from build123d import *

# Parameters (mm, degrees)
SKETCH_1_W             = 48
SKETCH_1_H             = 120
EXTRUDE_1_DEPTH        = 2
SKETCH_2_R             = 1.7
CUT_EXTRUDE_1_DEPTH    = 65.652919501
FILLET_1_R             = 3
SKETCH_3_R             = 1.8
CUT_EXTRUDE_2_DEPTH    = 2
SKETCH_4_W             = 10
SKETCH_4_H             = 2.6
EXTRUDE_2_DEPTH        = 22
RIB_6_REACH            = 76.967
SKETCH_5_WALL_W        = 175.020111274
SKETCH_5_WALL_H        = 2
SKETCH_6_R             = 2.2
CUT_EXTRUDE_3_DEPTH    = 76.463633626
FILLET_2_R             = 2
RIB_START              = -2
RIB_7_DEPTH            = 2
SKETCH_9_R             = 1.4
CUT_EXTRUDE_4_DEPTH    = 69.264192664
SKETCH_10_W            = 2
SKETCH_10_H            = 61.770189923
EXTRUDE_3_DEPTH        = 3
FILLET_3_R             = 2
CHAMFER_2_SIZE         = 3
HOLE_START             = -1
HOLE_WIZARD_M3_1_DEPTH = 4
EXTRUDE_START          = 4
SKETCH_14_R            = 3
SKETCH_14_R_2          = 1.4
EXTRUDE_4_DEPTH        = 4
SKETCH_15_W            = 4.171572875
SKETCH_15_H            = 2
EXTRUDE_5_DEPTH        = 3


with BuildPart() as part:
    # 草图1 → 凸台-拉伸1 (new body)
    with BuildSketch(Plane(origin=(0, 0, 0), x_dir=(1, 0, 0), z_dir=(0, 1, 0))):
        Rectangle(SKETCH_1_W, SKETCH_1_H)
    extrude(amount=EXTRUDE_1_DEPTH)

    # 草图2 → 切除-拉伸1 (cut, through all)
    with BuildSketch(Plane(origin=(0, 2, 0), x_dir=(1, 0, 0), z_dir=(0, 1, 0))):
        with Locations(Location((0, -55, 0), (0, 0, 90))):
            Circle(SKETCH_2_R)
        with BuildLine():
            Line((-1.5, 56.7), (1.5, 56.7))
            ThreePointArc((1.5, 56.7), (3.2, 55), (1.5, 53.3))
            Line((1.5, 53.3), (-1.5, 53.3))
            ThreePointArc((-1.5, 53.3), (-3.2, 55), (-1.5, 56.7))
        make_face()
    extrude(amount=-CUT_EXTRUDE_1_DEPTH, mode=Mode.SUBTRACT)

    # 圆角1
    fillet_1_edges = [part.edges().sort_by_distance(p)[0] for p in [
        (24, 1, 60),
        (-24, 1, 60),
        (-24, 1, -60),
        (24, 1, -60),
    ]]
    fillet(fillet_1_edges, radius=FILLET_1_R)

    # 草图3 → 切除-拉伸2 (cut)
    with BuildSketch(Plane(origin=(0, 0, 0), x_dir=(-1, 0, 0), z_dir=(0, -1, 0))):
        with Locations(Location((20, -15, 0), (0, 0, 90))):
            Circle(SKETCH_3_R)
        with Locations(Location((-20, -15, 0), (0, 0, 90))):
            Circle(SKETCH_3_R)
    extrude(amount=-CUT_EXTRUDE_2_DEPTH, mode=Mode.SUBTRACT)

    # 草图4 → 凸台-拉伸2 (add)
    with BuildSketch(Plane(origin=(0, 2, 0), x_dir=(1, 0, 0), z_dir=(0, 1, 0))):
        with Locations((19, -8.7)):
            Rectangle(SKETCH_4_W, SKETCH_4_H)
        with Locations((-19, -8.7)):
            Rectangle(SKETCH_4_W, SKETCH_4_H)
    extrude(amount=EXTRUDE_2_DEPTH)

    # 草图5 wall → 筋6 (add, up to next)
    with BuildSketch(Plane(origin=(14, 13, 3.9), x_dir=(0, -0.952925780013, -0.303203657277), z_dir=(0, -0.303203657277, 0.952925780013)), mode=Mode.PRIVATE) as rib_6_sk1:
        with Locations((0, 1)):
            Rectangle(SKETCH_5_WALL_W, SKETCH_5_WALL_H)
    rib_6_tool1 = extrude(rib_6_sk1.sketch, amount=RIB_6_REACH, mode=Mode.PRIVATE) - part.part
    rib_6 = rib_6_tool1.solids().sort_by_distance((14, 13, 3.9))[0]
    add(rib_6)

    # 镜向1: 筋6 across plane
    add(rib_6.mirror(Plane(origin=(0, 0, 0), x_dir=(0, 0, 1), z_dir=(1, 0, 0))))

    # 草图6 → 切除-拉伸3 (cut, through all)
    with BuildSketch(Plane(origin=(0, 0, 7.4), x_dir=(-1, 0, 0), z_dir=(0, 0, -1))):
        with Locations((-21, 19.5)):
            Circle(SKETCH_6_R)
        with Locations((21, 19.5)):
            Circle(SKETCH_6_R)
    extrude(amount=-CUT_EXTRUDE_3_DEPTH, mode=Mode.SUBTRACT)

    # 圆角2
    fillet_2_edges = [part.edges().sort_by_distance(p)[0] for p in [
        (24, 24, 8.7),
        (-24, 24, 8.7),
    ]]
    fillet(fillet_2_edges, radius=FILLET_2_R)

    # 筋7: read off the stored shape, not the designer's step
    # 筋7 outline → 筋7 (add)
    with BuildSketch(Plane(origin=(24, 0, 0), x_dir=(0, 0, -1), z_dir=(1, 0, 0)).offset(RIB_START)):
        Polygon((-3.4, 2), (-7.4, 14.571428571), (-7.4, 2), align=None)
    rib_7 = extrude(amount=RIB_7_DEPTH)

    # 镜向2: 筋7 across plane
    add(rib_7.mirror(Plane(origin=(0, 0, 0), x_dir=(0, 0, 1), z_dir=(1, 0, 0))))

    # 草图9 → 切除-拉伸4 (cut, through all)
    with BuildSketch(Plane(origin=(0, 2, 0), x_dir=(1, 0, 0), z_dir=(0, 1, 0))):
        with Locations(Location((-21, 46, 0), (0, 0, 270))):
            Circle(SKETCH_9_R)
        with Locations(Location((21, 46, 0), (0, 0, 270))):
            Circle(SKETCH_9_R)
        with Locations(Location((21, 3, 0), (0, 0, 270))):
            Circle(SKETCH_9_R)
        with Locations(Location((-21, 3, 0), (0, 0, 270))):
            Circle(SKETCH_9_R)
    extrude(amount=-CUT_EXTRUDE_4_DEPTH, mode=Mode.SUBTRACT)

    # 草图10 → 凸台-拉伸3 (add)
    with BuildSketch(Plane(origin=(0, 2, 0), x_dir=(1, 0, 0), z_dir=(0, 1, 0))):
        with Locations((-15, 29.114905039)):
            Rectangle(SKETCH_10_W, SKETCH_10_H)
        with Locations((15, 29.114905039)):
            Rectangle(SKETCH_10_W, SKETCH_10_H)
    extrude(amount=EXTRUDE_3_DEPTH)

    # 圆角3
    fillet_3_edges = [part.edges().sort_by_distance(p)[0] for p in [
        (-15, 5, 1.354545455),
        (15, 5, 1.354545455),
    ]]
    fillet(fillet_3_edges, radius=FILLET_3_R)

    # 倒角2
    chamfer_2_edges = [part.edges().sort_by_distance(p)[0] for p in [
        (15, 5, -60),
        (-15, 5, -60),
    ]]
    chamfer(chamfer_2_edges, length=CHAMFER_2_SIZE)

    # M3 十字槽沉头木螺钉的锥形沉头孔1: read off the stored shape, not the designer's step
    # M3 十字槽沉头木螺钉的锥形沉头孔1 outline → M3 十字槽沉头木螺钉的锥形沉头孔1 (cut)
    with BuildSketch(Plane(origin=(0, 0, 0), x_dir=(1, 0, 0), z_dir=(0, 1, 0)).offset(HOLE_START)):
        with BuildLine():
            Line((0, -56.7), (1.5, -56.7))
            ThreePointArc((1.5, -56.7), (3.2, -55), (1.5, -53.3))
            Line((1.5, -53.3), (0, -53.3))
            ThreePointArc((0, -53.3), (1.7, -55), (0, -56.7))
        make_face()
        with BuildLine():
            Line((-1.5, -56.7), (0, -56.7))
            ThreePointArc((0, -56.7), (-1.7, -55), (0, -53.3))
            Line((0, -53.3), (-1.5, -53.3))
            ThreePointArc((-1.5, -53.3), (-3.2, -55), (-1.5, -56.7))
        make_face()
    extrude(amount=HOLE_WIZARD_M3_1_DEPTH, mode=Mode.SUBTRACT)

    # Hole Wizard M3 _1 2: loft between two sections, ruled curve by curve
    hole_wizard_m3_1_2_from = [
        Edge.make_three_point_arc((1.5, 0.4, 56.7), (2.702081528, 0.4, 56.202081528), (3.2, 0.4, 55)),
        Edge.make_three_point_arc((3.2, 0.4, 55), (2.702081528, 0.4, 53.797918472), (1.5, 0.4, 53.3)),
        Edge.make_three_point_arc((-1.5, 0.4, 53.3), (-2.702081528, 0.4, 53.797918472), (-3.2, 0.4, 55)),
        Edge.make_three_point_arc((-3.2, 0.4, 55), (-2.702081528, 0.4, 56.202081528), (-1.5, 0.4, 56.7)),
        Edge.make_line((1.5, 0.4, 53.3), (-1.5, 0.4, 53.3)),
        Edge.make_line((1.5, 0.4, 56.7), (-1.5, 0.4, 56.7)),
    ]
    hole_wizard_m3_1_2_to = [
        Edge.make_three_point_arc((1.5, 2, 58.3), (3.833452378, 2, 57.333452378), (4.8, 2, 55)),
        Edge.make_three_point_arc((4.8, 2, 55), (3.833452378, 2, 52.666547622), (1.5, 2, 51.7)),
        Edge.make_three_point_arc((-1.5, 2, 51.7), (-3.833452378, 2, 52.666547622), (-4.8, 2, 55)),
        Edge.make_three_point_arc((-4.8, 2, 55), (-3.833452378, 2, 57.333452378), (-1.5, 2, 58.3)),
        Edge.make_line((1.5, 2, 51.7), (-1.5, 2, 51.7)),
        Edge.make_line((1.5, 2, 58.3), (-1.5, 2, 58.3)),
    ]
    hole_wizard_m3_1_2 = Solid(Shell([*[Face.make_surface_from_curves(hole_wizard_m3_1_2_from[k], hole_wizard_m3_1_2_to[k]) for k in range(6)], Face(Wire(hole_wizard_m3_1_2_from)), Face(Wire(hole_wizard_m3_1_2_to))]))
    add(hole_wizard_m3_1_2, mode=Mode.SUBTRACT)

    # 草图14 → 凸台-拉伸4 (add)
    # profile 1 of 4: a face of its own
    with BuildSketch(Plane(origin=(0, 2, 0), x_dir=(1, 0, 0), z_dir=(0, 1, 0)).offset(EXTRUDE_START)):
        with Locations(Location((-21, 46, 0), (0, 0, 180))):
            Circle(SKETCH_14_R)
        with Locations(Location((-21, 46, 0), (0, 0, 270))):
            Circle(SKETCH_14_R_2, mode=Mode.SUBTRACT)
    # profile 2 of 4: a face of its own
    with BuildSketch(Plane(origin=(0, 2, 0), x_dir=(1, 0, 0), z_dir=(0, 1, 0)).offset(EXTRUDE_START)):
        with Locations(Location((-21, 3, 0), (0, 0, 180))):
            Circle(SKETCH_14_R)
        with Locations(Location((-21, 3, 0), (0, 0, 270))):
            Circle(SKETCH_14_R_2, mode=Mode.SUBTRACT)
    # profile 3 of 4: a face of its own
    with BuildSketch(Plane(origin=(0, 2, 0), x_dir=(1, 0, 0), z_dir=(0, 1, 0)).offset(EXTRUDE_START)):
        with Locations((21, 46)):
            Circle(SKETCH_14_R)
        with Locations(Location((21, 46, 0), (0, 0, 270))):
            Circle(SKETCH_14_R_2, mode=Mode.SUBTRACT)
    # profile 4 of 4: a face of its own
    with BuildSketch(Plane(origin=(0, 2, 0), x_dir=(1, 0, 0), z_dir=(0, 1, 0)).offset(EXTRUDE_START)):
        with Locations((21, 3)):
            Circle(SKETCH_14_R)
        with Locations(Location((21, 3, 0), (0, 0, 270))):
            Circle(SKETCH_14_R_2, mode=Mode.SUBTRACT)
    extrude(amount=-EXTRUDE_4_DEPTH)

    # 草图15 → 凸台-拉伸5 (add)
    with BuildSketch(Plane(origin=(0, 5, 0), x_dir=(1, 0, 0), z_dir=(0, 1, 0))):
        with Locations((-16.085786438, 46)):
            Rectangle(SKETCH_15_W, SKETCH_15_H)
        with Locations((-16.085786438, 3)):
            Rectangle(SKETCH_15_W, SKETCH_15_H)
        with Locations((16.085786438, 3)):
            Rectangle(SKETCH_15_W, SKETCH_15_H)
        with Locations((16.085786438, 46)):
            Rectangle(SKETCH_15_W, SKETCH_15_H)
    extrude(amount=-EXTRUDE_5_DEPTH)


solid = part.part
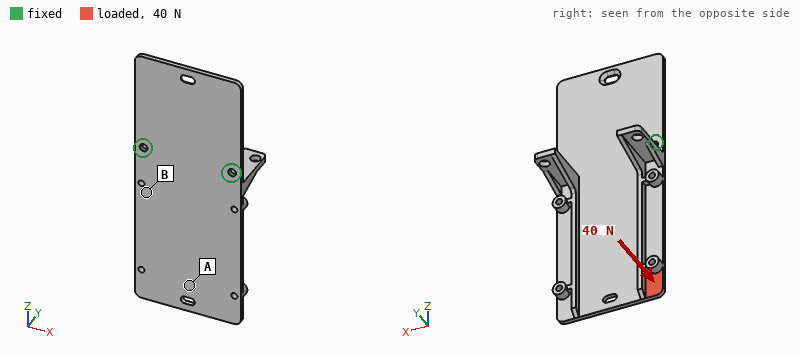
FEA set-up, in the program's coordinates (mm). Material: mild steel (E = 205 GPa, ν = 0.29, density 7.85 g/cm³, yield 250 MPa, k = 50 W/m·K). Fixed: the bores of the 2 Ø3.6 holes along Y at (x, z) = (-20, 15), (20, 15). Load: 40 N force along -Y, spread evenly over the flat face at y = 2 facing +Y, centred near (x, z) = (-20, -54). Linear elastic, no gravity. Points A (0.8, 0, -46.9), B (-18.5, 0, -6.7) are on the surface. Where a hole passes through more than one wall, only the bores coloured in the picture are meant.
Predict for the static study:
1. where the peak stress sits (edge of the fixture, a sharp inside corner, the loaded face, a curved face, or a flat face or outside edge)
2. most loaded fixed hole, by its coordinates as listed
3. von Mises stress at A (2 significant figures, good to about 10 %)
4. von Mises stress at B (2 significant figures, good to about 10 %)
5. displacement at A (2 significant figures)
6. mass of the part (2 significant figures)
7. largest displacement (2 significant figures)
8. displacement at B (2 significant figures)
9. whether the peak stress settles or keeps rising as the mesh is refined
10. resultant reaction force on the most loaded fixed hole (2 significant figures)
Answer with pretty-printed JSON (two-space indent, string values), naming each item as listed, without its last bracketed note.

{
  "where the peak stress sits": "edge of the fixture",
  "most loaded fixed hole, by its coordinates as listed": "(-20, 15)",
  "von Mises stress at A": "16 MPa",
  "von Mises stress at B": "36 MPa",
  "displacement at A": "0.29 mm",
  "mass of the part": "110 g",
  "largest displacement": "0.46 mm",
  "displacement at B": "0.081 mm",
  "whether the peak stress settles or keeps rising as the mesh is refined": "keeps rising",
  "resultant reaction force on the most loaded fixed hole": "37 N"
}
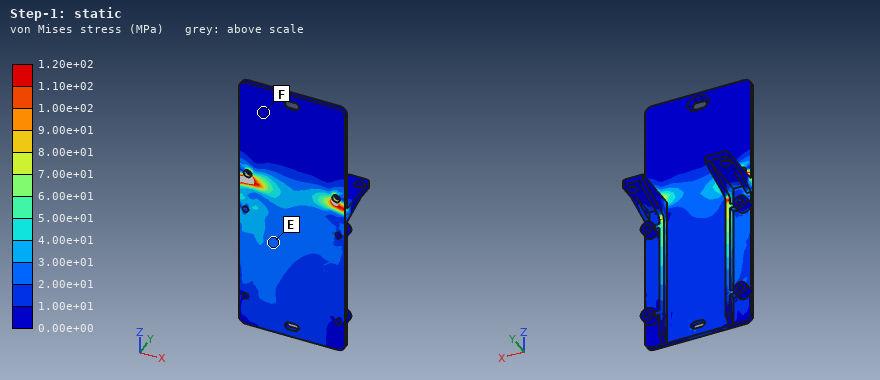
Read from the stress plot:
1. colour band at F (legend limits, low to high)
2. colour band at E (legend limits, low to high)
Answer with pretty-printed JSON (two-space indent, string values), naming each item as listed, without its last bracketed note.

{
  "colour band at F": "0.00e+00 to 1.00e+01 MPa",
  "colour band at E": "2.00e+01 to 3.00e+01 MPa"
}
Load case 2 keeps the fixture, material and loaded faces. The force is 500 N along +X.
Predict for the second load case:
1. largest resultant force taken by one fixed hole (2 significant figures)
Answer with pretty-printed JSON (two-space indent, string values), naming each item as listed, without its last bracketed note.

{
  "largest resultant force taken by one fixed hole": "880 N"
}
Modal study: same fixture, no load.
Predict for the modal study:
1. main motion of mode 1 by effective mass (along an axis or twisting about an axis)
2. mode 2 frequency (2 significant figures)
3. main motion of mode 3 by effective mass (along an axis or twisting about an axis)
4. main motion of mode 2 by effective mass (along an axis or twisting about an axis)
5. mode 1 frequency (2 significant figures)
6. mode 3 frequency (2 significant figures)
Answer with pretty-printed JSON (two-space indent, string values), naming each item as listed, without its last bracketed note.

{
  "main motion of mode 1 by effective mass": "along Y",
  "mode 2 frequency": "790 Hz",
  "main motion of mode 3 by effective mass": "twisting about Z",
  "main motion of mode 2 by effective mass": "along Y",
  "mode 1 frequency": "360 Hz",
  "mode 3 frequency": "1100 Hz"
}
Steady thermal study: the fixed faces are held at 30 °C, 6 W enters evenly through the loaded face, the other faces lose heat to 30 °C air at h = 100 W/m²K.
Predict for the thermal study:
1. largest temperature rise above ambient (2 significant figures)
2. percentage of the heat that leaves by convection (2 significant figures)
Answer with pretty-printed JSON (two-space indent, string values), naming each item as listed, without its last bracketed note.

{
  "largest temperature rise above ambient": "47 K",
  "percentage of the heat that leaves by convection": "96 %"
}
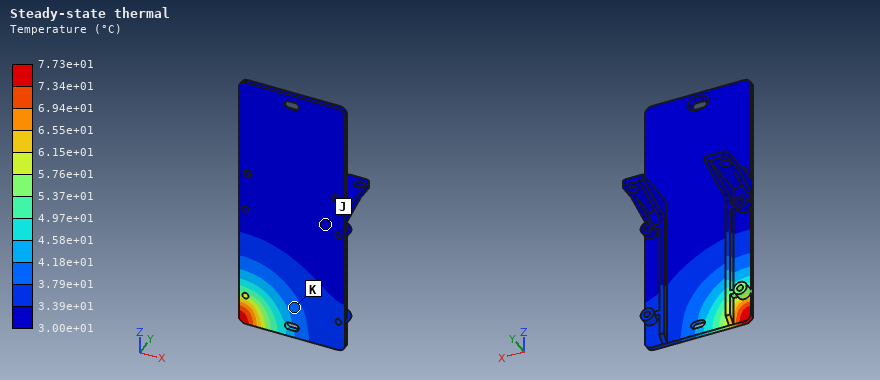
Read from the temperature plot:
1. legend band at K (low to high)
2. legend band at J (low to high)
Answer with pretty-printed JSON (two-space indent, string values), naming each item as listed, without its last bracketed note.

{
  "legend band at K": "3.79e+01 to 4.18e+01 °C",
  "legend band at J": "3.00e+01 to 3.39e+01 °C"
}
